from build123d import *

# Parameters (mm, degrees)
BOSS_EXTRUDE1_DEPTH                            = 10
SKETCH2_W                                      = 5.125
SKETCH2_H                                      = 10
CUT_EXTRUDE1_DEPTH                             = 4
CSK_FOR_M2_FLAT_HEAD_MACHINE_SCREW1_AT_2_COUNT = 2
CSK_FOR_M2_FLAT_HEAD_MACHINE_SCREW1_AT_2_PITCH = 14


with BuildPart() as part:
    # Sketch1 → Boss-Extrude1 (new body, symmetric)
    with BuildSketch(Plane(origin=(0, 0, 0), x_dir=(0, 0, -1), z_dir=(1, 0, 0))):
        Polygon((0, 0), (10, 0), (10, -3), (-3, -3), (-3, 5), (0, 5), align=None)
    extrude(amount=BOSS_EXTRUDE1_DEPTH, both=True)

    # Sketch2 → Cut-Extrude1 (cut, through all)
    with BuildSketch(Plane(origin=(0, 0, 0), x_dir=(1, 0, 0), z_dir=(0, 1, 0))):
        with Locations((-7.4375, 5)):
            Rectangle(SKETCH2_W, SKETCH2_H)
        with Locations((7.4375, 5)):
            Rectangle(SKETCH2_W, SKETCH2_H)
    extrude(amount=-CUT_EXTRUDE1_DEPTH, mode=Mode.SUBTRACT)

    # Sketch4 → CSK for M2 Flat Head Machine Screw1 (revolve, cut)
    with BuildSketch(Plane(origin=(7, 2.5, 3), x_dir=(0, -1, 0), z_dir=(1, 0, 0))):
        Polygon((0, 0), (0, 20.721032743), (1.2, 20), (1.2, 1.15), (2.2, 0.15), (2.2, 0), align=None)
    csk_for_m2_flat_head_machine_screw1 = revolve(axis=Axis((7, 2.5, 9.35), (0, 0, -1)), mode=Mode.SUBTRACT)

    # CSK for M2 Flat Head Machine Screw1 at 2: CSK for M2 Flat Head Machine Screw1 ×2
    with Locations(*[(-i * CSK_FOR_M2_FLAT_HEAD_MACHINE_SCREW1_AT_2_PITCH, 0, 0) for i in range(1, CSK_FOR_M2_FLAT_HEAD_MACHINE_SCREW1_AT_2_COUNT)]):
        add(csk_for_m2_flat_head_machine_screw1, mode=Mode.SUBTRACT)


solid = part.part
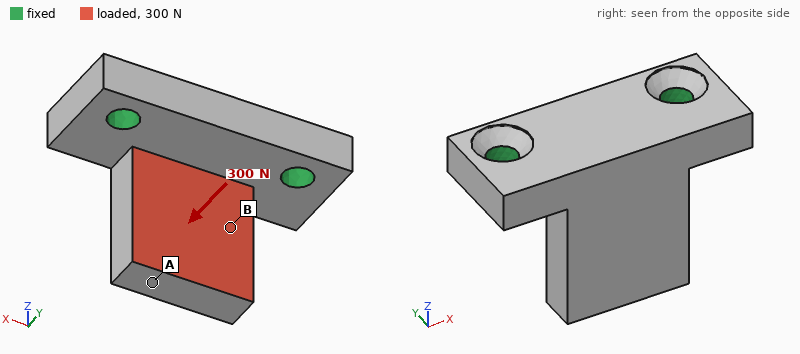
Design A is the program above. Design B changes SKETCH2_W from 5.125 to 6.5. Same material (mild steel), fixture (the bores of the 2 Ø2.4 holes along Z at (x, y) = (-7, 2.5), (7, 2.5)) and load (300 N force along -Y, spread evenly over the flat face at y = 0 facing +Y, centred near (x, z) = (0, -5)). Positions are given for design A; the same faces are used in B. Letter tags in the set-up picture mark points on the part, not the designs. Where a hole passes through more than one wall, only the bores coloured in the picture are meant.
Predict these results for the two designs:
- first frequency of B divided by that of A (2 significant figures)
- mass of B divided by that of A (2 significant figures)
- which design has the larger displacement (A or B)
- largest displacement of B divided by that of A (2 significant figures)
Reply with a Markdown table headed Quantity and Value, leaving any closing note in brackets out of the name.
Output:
| Quantity | Value |
|---|---|
| first frequency of B divided by that of A | 1.0 |
| mass of B divided by that of A | 0.94 |
| which design has the larger displacement | B |
| largest displacement of B divided by that of A | 1.1 |
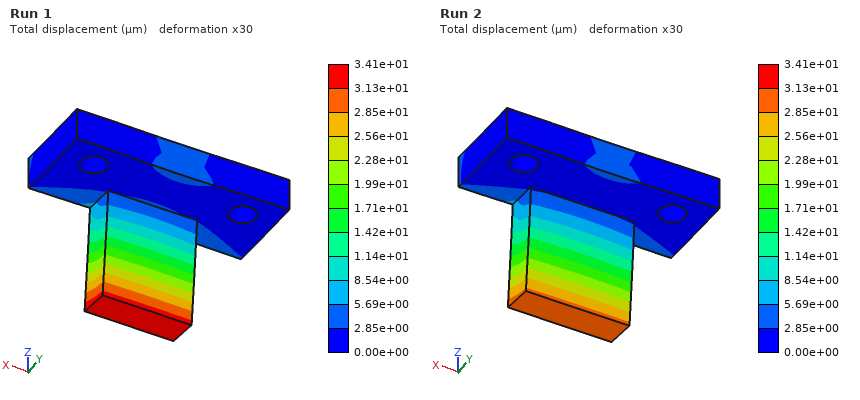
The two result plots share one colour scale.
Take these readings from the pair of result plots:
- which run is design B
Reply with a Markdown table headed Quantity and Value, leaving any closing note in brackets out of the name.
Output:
| Quantity | Value |
|---|---|
| which run is design B | Run 1 |
